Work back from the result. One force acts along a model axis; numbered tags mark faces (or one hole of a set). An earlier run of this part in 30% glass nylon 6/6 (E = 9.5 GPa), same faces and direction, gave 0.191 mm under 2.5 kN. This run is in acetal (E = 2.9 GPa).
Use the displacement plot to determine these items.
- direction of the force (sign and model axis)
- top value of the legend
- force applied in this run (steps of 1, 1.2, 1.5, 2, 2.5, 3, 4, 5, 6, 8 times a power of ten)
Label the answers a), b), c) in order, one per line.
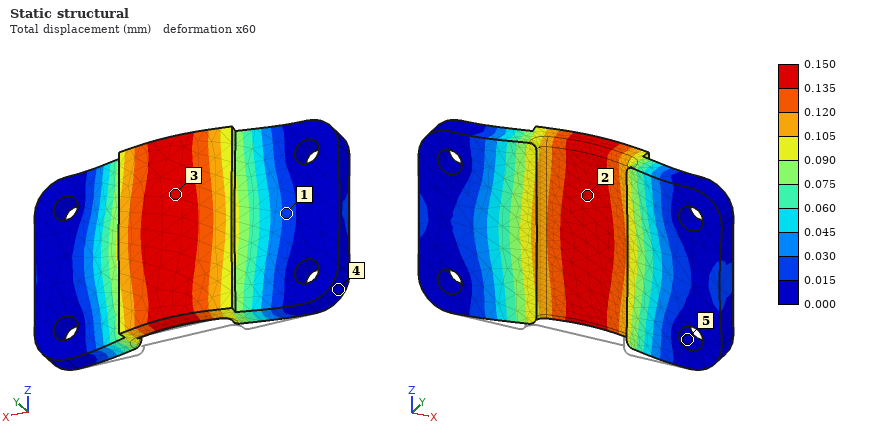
a) +Y
b) 0.150 mm
c) 600 N
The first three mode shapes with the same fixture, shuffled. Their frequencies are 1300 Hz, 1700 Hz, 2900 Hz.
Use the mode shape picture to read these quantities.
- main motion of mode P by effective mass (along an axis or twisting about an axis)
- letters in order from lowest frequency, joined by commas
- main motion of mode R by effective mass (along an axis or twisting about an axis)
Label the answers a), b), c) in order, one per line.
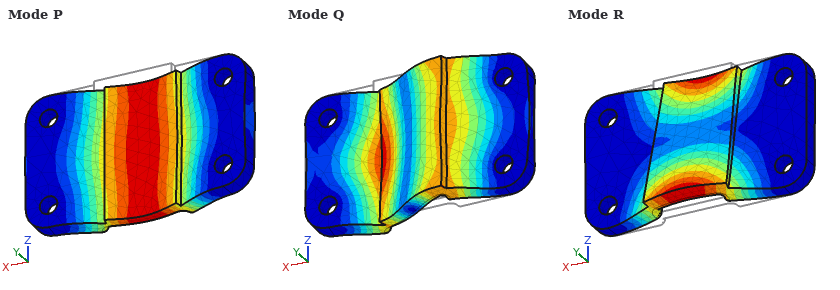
a) along Y
b) P, R, Q
c) twisting about X
